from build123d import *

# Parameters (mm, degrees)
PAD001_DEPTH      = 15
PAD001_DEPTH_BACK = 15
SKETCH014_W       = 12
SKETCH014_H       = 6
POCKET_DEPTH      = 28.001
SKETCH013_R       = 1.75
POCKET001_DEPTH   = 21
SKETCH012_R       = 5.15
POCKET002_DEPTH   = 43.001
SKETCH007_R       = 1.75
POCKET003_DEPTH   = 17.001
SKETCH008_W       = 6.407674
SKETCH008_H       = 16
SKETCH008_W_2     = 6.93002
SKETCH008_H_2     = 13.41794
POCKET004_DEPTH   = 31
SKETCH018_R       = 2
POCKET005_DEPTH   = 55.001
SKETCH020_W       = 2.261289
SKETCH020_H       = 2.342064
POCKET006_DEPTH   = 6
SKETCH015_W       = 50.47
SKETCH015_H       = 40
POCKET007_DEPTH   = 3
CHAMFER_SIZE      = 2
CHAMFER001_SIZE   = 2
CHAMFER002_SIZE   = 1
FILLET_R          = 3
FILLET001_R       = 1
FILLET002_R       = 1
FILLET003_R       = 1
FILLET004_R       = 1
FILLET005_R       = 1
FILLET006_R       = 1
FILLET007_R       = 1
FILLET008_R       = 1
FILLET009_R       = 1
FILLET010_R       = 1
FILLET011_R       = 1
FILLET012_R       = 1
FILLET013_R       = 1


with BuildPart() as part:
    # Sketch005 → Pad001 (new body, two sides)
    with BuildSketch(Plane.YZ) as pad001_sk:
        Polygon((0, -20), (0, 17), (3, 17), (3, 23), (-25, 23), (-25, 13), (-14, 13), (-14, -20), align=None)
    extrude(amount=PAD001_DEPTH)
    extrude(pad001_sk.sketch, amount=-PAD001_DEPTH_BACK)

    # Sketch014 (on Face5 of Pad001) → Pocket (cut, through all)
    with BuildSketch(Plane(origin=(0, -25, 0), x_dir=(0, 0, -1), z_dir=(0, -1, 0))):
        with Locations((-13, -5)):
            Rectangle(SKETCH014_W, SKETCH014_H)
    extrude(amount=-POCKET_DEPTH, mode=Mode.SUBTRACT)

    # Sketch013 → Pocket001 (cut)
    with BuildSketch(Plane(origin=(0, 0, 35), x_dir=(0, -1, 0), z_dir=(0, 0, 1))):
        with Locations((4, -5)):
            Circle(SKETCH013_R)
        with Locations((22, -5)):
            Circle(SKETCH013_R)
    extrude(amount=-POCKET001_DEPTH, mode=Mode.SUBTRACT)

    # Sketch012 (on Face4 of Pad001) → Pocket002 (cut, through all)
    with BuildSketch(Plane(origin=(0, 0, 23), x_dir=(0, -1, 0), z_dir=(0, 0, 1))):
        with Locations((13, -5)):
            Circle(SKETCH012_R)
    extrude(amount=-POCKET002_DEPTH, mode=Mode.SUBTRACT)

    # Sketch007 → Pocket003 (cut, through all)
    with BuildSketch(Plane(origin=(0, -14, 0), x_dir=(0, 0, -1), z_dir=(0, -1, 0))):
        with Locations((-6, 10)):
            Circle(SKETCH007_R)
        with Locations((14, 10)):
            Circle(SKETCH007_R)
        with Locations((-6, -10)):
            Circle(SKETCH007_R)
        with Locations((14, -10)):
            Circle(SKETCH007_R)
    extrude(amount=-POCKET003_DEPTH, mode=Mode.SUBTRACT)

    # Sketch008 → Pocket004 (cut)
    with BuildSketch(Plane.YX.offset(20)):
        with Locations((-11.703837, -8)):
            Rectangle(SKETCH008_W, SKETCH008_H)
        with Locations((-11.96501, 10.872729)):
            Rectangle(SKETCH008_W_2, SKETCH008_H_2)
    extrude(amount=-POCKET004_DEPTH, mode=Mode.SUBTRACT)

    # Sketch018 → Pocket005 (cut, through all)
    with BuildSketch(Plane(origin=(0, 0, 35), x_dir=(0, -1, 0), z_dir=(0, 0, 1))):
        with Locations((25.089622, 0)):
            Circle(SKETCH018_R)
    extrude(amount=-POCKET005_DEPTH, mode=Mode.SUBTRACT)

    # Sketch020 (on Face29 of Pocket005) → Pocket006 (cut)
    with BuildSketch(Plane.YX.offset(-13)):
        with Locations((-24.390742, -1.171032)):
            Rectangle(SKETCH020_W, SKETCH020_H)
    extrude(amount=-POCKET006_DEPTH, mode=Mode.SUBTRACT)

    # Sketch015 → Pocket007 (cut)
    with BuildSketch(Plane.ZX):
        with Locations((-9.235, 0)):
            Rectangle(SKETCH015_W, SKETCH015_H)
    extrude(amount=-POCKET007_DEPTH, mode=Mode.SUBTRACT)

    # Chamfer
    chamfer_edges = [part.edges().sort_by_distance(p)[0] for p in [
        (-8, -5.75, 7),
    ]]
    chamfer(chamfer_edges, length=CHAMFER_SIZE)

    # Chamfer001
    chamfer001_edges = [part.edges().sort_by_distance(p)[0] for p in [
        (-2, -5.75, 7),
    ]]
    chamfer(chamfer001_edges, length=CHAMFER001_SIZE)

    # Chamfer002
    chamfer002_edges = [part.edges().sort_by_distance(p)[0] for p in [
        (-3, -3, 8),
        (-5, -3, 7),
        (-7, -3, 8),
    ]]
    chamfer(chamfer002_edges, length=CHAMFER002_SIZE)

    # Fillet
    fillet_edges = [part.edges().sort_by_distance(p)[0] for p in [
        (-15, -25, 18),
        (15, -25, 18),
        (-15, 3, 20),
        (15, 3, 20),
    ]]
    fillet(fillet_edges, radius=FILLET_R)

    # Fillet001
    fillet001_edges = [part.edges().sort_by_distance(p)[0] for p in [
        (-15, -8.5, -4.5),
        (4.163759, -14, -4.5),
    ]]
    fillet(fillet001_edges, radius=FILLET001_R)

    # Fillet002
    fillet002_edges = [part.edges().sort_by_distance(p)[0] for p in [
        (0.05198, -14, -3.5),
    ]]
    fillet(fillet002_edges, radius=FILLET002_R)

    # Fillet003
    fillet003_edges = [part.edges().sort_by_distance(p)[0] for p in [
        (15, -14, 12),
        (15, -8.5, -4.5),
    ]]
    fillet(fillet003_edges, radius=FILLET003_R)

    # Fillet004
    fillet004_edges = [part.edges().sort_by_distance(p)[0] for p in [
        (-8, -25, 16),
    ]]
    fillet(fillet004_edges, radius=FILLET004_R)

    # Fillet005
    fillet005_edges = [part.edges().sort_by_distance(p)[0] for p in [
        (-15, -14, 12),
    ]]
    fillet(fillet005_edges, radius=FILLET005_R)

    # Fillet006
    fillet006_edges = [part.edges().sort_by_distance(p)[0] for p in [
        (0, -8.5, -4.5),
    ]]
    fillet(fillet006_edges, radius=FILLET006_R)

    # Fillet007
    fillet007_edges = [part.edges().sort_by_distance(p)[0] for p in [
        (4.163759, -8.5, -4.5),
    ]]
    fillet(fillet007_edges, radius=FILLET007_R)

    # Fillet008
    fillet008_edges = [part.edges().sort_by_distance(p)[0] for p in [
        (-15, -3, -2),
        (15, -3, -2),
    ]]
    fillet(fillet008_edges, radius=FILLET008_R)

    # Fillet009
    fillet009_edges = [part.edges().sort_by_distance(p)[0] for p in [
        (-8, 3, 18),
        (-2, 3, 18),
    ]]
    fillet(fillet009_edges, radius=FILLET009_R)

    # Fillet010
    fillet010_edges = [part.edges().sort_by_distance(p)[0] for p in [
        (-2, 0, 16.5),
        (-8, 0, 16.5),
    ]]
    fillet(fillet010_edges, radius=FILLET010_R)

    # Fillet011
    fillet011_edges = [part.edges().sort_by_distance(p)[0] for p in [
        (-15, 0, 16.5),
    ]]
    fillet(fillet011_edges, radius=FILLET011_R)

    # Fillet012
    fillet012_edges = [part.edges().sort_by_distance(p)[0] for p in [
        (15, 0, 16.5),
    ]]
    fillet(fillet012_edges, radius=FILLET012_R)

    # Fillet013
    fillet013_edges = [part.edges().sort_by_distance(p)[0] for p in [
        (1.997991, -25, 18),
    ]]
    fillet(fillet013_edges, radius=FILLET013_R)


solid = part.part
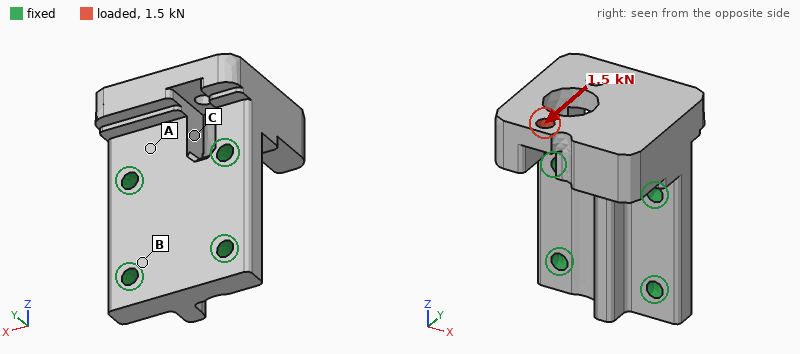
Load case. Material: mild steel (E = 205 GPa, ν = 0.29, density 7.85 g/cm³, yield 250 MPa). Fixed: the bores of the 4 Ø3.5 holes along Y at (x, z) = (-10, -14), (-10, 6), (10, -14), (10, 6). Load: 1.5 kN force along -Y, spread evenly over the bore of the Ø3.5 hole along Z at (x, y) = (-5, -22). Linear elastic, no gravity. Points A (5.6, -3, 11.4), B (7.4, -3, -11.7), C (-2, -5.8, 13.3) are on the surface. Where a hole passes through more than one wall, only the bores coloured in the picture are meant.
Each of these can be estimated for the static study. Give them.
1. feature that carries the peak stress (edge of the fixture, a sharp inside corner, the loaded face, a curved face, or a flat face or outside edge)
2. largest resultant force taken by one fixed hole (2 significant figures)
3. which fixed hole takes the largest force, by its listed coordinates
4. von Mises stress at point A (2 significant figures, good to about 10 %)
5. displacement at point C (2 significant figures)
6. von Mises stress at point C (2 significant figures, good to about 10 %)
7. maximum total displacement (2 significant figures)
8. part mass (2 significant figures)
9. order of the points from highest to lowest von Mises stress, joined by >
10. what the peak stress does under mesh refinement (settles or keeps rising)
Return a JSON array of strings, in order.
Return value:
["edge of the fixture", "1.1 kN", "(-10, 6)", "52 MPa", "8.3 µm", "26 MPa", "40 µm", "95 g", "A > C > B", "keeps rising"]
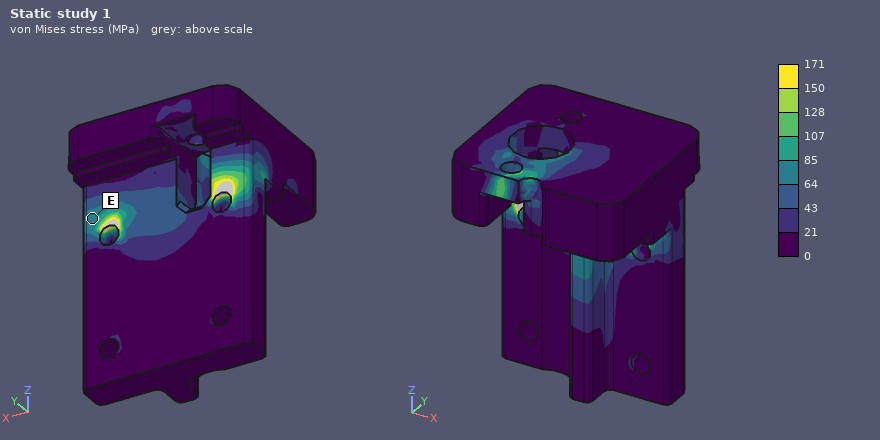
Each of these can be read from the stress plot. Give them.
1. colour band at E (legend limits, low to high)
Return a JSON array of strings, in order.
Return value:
["64 to 85 MPa"]
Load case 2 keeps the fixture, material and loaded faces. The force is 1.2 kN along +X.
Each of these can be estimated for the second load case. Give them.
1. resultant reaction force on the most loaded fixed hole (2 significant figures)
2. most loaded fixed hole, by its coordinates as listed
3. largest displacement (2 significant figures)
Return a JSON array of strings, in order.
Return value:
["1.4 kN", "(10, 6)", "17 µm"]
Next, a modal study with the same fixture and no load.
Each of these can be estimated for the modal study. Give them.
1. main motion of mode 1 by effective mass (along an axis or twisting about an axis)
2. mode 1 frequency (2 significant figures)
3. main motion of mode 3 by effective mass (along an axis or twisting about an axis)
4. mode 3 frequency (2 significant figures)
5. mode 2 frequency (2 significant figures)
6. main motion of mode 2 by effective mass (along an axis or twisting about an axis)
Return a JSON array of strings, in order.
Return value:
["along Y", "6200 Hz", "along X", "14 kHz", "10 kHz", "along X"]
